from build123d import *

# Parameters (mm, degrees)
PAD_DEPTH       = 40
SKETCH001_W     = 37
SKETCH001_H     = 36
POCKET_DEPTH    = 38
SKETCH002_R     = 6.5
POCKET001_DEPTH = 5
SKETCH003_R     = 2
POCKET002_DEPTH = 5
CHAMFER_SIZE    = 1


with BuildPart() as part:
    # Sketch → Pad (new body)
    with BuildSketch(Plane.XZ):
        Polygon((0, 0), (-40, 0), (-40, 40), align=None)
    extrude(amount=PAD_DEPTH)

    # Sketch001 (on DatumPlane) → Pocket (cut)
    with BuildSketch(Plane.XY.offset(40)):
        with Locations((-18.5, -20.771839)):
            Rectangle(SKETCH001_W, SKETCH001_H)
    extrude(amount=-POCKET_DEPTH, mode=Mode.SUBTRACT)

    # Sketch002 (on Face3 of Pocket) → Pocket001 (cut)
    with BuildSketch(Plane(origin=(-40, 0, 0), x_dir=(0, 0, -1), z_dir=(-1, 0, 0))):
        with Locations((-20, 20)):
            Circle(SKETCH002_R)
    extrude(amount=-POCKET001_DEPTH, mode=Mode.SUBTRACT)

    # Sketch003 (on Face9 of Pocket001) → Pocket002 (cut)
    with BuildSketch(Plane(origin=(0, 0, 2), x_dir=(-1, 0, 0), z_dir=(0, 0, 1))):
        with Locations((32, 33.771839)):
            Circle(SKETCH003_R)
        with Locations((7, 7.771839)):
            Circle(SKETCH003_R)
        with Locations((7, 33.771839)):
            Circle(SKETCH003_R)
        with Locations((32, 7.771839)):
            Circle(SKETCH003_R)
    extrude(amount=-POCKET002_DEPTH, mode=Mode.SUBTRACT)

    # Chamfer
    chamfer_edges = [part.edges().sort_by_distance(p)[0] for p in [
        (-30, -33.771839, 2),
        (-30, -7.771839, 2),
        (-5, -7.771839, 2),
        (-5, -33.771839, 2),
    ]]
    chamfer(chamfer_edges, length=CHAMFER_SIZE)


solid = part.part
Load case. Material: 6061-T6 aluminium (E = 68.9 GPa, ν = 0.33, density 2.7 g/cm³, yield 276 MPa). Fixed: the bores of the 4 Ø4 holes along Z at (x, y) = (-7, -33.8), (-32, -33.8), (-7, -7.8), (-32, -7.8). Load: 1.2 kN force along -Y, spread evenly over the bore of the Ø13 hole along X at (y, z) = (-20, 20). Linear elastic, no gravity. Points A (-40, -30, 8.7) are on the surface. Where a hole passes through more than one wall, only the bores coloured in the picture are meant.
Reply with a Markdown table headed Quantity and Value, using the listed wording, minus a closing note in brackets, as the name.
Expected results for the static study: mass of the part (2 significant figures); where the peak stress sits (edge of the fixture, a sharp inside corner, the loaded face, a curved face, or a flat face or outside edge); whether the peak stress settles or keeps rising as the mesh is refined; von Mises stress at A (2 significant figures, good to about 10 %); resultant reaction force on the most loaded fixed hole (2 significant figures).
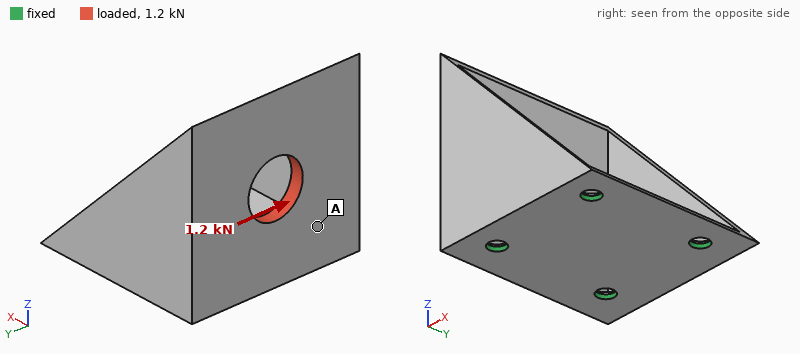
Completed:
| Quantity | Value |
|---|---|
| mass of the part | 25 g |
| where the peak stress sits | edge of the fixture |
| whether the peak stress settles or keeps rising as the mesh is refined | keeps rising |
| von Mises stress at A | 18 MPa |
| resultant reaction force on the most loaded fixed hole | 1.1 kN |
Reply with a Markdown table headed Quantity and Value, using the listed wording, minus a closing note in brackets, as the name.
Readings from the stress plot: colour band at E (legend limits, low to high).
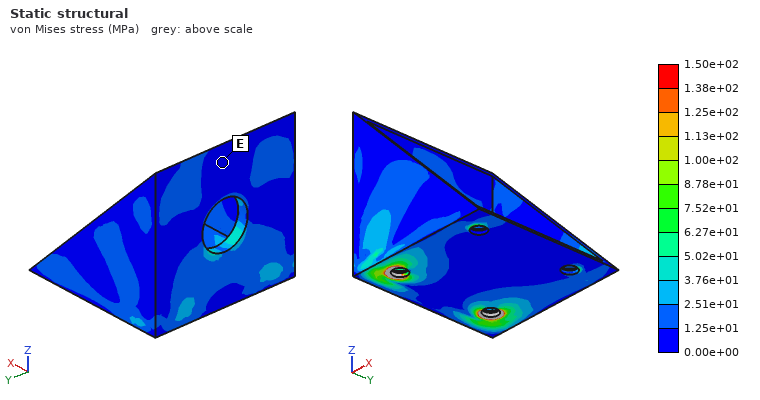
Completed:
| Quantity | Value |
|---|---|
| colour band at E | 0.00e+00 to 1.25e+01 MPa |
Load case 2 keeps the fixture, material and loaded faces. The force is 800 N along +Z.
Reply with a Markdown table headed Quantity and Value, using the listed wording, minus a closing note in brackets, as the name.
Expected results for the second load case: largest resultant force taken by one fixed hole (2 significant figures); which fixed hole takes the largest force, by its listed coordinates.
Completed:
| Quantity | Value |
|---|---|
| largest resultant force taken by one fixed hole | 510 N |
| which fixed hole takes the largest force, by its listed coordinates | (-32, -7.8) |
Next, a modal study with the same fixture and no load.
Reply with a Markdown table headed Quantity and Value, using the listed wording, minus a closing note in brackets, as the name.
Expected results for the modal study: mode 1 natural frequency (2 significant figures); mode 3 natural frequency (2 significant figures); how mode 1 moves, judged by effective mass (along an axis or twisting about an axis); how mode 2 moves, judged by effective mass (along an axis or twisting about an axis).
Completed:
| Quantity | Value |
|---|---|
| mode 1 natural frequency | 3900 Hz |
| mode 3 natural frequency | 6200 Hz |
| how mode 1 moves, judged by effective mass | along X |
| how mode 2 moves, judged by effective mass | along Y |
